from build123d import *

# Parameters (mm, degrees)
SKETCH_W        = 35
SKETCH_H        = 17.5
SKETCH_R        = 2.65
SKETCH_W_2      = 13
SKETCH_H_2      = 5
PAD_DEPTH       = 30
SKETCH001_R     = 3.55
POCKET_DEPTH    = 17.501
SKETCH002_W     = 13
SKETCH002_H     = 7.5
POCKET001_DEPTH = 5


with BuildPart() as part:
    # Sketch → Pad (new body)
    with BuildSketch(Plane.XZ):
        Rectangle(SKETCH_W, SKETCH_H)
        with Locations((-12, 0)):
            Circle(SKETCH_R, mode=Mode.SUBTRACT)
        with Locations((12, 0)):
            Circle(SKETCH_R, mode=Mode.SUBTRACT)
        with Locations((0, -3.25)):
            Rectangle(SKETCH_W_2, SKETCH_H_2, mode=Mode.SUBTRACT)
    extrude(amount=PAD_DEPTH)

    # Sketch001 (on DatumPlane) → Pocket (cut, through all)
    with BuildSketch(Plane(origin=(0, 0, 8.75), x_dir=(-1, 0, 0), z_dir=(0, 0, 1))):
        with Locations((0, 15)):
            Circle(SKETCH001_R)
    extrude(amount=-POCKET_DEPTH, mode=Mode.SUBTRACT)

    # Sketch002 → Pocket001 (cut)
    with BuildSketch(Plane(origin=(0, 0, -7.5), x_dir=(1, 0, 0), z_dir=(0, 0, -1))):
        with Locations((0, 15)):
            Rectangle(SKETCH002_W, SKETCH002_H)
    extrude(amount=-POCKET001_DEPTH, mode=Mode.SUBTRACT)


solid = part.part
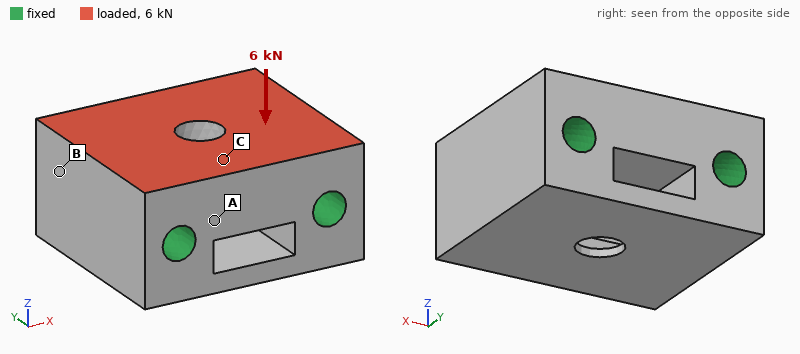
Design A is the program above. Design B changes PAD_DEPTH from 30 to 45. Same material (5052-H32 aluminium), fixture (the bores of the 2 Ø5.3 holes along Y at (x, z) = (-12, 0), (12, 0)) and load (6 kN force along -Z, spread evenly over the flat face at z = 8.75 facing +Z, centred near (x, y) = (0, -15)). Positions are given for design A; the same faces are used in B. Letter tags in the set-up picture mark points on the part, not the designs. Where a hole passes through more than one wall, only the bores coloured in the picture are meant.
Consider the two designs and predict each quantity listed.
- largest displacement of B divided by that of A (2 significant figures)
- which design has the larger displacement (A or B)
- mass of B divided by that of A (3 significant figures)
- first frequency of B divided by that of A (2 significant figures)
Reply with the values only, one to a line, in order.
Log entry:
0.67
A
1.52
1.0
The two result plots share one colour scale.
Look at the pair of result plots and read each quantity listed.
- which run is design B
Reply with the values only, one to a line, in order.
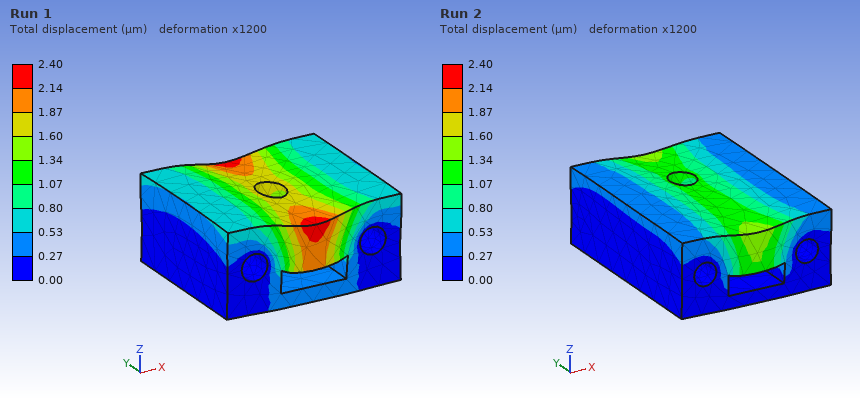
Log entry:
Run 2
